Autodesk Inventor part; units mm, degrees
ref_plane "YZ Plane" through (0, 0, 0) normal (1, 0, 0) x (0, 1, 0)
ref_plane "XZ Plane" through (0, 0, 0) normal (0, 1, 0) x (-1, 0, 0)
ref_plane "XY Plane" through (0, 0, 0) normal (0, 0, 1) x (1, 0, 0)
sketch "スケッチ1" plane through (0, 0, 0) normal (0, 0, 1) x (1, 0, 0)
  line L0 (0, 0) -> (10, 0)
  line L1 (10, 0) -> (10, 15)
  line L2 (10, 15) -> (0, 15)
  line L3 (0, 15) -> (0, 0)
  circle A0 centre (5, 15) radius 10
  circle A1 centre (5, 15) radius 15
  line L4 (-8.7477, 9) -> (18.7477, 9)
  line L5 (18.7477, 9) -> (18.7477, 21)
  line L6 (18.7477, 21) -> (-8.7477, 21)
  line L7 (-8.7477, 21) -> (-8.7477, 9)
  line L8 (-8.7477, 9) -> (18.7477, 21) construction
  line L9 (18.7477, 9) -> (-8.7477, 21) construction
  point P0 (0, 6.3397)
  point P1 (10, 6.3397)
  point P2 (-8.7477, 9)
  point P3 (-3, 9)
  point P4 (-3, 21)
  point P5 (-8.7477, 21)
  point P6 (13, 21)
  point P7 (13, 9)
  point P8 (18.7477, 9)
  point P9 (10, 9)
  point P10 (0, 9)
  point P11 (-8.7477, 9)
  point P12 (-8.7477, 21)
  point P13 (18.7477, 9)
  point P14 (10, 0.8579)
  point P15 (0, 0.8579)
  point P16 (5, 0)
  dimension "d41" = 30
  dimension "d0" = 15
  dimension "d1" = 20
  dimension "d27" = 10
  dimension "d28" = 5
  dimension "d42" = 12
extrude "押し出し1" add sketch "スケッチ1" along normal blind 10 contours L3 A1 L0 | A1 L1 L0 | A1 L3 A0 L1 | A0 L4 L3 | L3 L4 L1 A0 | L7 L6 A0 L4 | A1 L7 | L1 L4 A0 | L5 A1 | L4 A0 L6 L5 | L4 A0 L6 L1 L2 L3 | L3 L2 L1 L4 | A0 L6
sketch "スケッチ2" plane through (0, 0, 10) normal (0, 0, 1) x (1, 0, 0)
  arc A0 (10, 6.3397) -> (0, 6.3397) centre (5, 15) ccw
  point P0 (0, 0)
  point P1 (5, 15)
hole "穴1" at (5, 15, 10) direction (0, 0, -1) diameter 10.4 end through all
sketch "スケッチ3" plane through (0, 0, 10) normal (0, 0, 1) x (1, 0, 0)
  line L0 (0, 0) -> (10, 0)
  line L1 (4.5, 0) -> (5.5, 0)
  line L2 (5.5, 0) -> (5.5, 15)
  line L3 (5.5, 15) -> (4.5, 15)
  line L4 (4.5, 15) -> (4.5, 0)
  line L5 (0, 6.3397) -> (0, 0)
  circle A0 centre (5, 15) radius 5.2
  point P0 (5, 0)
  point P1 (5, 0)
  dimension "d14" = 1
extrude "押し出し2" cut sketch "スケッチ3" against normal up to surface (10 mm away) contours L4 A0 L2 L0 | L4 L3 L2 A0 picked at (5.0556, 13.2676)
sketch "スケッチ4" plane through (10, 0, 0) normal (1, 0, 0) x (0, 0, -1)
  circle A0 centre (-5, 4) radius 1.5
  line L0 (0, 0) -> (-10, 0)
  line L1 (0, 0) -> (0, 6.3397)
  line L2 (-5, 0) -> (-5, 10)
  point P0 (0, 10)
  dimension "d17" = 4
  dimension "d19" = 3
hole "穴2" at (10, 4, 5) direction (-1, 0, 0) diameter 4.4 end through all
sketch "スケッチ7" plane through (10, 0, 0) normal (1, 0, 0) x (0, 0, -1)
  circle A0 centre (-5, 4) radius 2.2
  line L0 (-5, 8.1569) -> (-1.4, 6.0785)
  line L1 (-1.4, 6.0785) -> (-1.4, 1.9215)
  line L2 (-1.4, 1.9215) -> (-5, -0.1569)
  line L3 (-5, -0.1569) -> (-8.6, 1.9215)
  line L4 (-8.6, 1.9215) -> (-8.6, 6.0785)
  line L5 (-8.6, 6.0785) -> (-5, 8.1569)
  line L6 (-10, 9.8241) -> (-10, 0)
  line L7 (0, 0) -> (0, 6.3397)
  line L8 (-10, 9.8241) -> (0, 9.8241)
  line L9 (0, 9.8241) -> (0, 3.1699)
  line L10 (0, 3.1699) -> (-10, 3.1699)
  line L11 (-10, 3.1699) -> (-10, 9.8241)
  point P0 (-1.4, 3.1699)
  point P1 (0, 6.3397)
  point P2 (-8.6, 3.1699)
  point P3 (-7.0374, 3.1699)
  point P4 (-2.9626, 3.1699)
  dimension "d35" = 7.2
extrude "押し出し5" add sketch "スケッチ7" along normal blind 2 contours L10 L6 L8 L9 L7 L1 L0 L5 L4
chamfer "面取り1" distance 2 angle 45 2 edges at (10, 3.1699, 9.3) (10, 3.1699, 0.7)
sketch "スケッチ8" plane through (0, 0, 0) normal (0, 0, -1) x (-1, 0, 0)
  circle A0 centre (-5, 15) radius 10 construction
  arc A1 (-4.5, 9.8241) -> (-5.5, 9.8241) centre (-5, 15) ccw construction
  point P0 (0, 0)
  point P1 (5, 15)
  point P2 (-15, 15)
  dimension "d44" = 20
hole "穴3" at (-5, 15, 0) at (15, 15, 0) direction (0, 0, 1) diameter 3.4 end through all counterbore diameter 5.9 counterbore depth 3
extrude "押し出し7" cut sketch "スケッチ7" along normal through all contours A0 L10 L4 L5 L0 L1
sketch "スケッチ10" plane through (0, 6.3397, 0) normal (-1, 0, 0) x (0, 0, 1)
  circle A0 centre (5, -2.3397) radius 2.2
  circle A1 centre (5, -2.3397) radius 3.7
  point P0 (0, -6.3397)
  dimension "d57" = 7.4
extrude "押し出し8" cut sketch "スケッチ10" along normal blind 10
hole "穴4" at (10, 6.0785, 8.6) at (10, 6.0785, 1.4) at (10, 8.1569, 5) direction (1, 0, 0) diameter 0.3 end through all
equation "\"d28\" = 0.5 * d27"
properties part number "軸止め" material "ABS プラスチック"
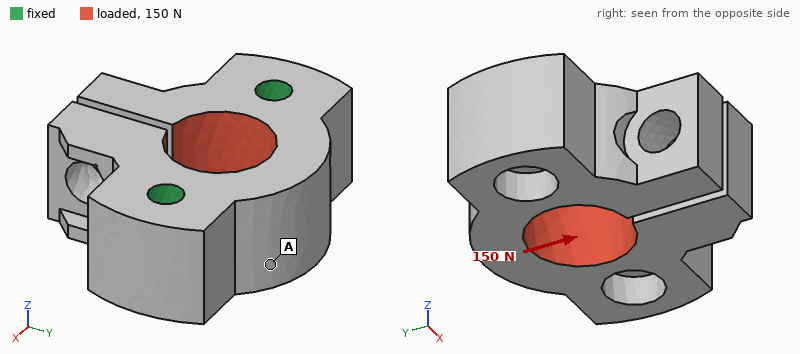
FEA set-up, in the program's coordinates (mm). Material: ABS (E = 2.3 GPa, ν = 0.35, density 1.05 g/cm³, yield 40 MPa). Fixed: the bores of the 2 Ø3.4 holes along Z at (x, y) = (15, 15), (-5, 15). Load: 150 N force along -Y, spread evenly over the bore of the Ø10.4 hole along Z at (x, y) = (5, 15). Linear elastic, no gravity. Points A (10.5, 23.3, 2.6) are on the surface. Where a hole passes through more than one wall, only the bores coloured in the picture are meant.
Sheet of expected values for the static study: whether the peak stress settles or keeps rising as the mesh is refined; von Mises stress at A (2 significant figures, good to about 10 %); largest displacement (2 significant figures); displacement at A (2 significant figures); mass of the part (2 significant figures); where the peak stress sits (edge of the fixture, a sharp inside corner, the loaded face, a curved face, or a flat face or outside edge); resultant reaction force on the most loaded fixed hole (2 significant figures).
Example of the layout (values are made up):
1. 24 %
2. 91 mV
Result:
1. keeps rising
2. 1.1 MPa
3. 47 µm
4. 9.4 µm
5. 3.8 g
6. edge of the fixture
7. 83 N
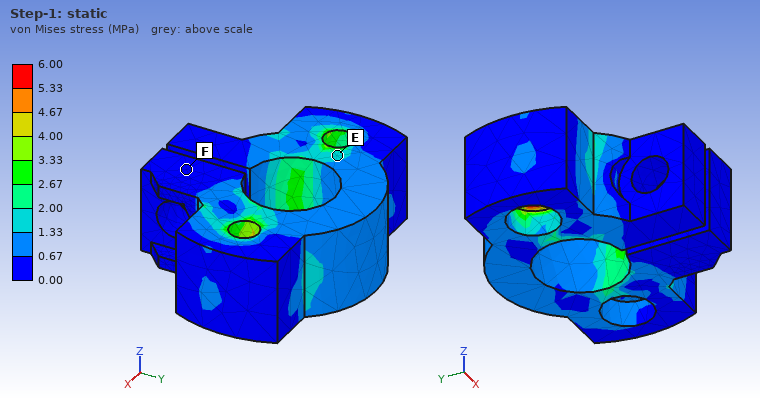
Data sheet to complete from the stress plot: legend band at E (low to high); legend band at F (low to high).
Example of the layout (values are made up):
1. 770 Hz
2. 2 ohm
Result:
1. 1.33 to 2.00 MPa
2. 0.00 to 0.67 MPa
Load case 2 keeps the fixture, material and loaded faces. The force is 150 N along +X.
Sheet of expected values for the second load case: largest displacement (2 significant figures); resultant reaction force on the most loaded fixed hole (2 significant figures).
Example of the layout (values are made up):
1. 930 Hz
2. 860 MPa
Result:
1. 7.1 µm
2. 75 N
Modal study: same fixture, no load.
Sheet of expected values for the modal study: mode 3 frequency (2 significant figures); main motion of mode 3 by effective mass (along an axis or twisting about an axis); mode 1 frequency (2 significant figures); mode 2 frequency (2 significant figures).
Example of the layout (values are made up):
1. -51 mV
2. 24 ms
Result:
1. 6300 Hz
2. along Z
3. 5300 Hz
4. 5300 Hz
